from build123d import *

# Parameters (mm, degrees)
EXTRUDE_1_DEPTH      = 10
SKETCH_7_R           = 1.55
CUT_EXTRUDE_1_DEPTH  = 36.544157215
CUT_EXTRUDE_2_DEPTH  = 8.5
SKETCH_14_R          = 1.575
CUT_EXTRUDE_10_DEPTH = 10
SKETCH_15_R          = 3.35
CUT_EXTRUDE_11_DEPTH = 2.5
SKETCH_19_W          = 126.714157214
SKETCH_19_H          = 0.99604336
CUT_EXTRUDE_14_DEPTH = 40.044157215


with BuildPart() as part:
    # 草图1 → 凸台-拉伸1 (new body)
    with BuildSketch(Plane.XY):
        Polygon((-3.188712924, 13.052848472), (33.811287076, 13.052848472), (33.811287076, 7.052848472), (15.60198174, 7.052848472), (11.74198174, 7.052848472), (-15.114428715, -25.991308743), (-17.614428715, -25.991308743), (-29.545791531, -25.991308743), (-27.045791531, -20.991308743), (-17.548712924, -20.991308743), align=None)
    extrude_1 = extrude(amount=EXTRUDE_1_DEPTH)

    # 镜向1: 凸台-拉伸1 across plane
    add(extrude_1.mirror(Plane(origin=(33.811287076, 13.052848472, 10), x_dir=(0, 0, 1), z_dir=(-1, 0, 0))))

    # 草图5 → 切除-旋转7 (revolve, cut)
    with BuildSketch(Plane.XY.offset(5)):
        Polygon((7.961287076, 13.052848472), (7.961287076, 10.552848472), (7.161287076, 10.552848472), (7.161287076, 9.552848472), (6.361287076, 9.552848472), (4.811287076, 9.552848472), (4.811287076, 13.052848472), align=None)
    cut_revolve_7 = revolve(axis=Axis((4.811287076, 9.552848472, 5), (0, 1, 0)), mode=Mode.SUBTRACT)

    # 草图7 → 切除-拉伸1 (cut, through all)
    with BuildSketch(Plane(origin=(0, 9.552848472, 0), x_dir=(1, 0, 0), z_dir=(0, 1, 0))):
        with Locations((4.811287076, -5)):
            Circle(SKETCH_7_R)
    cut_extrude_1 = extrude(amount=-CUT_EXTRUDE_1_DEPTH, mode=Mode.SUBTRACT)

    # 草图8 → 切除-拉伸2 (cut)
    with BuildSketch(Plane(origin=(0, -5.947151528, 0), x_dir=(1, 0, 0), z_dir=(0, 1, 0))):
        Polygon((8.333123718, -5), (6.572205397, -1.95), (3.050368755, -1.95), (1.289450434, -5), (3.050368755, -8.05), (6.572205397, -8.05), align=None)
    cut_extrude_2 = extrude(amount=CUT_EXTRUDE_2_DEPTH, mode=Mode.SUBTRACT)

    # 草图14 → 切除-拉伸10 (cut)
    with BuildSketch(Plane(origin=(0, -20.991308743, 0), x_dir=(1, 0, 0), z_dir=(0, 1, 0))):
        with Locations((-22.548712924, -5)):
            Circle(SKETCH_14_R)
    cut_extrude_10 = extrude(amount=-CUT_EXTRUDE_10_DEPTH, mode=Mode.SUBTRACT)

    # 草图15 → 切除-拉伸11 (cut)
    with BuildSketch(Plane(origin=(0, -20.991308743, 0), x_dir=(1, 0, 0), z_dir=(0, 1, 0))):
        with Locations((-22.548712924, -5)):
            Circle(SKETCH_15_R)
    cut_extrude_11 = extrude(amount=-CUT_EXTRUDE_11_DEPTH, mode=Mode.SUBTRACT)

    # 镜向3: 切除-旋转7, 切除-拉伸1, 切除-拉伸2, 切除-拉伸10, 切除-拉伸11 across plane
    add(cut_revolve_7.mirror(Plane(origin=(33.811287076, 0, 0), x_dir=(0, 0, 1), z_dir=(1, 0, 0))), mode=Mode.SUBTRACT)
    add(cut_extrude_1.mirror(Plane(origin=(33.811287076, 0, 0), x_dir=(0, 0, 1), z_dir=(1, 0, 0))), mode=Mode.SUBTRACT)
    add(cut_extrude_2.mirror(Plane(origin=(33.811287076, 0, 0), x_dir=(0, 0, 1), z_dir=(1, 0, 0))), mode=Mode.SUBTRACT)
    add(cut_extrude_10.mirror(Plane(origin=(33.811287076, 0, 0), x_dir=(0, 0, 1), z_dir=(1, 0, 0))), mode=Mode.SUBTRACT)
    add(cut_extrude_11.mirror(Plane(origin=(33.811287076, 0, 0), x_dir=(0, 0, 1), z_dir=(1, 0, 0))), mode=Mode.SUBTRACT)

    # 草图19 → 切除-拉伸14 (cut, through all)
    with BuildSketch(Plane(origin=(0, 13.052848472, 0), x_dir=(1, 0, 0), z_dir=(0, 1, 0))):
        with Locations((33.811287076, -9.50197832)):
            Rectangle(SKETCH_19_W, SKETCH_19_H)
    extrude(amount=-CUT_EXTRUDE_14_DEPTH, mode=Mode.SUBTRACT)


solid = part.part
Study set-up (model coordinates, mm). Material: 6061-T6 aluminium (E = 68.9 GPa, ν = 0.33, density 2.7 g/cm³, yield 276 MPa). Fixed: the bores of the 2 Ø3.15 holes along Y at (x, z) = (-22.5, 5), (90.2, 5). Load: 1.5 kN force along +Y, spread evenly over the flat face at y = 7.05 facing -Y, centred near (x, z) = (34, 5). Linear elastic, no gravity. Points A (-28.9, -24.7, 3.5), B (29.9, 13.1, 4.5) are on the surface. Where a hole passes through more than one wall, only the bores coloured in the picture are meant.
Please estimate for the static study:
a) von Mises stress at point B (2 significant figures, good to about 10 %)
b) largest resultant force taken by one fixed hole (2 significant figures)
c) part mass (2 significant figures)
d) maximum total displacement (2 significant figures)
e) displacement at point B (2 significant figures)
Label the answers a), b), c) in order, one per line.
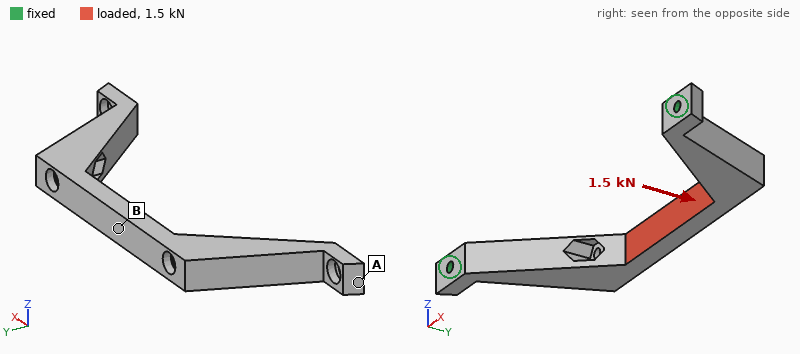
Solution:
a) 94 MPa
b) 1.1 kN
c) 29 g
d) 0.12 mm
e) 0.11 mm
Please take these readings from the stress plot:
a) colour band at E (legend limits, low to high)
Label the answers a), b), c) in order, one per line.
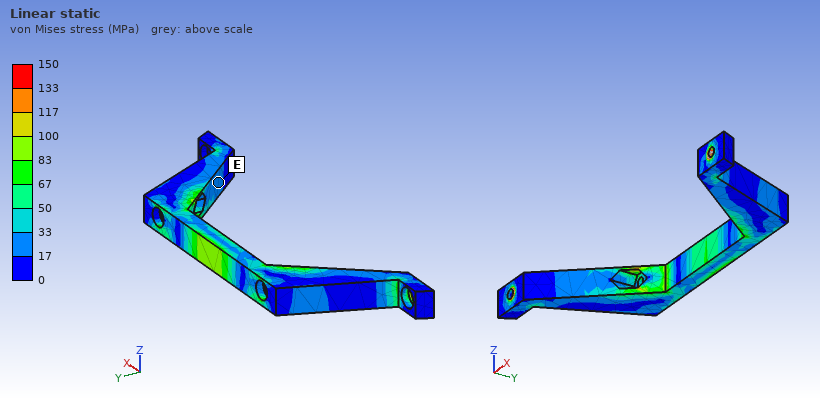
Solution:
a) 17 to 33 MPa
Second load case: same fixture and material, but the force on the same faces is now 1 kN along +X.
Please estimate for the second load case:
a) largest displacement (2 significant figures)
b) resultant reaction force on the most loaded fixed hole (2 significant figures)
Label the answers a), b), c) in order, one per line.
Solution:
a) 0.19 mm
b) 560 N
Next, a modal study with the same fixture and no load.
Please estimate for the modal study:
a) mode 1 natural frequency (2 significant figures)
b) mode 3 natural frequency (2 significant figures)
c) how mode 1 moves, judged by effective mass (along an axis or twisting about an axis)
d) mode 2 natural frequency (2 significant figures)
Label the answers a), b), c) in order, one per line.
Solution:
a) 1100 Hz
b) 2700 Hz
c) along Z
d) 2700 Hz
